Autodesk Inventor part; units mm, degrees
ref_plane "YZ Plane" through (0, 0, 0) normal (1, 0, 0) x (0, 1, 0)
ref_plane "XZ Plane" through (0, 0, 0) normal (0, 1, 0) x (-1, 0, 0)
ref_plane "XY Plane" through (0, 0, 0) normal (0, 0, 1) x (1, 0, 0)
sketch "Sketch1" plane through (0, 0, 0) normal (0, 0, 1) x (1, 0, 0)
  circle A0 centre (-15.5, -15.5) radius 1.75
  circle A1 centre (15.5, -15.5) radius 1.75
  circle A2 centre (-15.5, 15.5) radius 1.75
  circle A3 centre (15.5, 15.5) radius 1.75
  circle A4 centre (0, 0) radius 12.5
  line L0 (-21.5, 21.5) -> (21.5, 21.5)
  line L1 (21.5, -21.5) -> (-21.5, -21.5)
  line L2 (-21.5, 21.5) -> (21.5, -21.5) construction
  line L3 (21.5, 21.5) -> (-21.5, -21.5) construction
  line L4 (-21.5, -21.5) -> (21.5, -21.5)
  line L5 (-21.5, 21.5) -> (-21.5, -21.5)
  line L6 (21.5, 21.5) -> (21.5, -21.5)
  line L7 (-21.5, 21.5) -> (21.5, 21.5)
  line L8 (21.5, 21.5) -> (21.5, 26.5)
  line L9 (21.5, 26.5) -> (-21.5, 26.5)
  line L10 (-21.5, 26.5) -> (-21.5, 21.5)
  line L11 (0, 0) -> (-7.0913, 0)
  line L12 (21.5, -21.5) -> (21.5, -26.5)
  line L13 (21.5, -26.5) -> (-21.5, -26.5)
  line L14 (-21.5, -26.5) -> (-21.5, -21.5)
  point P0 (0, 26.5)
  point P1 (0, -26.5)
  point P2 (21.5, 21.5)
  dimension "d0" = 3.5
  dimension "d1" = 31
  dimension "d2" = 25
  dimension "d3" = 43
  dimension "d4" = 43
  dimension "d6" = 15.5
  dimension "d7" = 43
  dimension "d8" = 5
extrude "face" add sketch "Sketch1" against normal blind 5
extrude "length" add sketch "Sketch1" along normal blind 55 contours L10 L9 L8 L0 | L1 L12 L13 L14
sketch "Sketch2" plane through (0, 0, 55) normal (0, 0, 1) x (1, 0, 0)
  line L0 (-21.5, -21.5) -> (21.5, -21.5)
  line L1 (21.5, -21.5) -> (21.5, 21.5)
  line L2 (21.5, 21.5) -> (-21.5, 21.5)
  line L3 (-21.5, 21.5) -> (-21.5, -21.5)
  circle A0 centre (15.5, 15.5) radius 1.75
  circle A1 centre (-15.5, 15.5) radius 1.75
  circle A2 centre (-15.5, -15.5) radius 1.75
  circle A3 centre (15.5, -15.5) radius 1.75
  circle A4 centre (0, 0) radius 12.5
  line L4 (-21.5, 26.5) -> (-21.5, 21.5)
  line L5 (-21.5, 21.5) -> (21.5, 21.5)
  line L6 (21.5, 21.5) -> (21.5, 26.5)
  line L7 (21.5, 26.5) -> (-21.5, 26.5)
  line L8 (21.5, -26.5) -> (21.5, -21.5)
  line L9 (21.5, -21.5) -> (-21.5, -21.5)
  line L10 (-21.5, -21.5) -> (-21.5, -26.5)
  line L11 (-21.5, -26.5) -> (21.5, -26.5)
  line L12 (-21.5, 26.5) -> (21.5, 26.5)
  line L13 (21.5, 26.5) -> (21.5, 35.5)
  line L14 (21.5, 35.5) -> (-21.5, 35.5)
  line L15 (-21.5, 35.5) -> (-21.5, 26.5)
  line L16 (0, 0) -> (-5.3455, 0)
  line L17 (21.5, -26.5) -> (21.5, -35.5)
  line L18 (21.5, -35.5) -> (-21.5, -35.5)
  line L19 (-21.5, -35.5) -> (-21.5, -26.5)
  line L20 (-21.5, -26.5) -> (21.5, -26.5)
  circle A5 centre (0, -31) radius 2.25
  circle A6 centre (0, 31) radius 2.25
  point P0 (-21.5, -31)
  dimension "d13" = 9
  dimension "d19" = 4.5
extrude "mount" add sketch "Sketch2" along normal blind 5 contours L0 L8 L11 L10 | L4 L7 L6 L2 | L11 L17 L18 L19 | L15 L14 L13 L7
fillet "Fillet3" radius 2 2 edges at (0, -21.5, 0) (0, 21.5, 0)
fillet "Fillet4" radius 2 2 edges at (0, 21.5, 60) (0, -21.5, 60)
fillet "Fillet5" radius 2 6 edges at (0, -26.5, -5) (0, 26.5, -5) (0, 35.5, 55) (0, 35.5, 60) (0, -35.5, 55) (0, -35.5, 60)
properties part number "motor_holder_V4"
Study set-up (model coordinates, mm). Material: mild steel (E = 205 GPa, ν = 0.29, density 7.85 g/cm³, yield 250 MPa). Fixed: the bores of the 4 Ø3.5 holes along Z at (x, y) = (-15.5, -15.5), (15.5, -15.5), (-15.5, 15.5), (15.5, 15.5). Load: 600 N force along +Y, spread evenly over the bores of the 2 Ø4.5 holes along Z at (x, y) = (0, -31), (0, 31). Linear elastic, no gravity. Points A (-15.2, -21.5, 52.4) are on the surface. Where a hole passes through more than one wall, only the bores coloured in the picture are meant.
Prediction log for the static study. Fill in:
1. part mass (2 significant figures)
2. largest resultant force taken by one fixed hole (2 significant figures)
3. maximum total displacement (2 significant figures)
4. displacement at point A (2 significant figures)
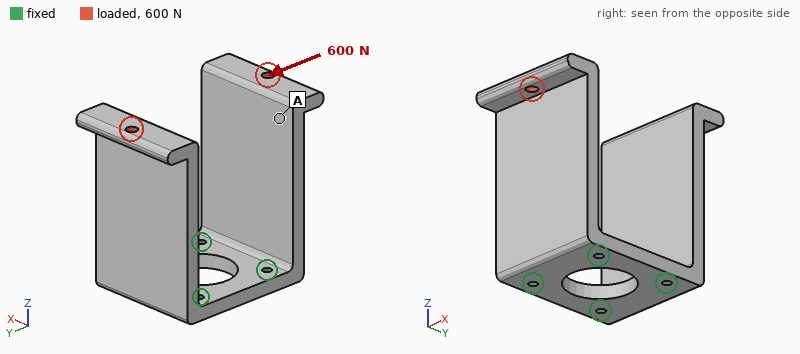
300 g
200 N
0.34 mm
0.27 mm
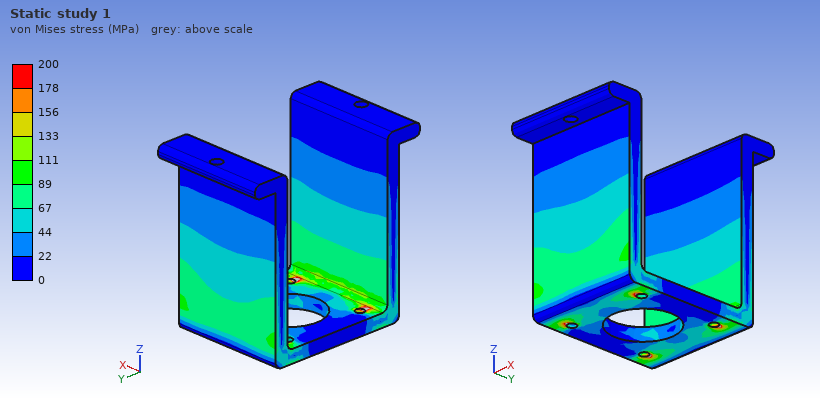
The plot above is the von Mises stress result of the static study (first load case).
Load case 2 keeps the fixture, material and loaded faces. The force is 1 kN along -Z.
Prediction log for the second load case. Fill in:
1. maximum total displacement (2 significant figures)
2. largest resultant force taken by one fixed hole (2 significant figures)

0.11 mm
250 N
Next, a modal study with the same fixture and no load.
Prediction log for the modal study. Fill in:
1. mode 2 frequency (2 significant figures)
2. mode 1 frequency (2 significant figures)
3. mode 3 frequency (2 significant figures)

740 Hz
730 Hz
2700 Hz
